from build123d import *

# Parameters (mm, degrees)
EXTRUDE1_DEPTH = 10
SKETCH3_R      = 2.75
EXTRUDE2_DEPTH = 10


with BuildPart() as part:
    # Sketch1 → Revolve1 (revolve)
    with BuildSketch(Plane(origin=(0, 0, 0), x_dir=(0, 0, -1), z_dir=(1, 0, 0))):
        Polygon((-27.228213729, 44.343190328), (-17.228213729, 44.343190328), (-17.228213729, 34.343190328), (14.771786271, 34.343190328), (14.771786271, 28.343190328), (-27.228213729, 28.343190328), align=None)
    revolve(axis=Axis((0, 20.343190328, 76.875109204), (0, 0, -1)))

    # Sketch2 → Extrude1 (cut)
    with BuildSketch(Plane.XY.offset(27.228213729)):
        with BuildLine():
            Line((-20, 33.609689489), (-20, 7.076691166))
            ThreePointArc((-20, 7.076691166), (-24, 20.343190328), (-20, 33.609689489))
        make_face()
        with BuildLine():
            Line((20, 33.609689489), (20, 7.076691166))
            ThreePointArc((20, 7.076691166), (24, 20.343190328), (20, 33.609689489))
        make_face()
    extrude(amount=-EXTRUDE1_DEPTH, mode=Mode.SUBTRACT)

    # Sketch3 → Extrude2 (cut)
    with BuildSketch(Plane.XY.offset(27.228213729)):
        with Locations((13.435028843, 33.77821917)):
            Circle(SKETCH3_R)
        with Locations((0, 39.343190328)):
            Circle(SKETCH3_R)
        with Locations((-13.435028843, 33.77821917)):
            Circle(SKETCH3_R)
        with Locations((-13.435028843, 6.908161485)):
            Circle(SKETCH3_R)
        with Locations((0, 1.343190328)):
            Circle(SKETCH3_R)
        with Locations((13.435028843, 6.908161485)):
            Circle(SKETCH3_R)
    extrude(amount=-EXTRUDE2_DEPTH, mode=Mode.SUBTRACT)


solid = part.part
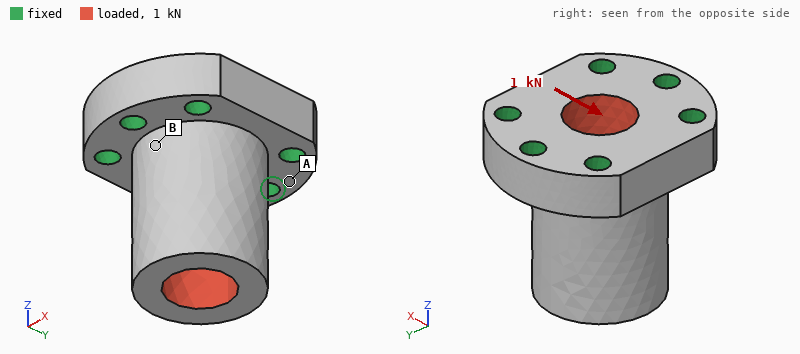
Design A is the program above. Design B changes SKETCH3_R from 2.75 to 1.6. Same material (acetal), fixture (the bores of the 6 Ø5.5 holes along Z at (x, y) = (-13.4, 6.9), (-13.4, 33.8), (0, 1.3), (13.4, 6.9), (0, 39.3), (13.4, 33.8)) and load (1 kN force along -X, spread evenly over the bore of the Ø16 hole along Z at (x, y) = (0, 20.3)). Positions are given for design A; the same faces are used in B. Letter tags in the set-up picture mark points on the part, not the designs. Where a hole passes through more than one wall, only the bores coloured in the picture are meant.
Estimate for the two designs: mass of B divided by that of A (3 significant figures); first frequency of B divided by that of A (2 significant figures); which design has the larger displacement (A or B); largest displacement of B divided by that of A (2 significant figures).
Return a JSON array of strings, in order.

["1.04", "0.94", "B", "1.1"]
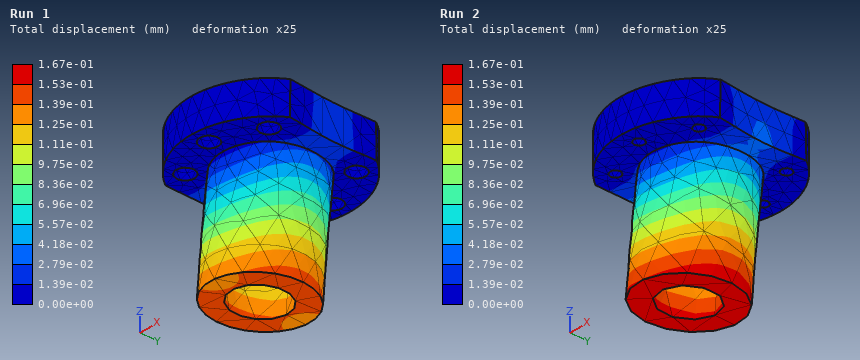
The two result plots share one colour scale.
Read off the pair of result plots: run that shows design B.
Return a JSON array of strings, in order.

["Run 2"]
